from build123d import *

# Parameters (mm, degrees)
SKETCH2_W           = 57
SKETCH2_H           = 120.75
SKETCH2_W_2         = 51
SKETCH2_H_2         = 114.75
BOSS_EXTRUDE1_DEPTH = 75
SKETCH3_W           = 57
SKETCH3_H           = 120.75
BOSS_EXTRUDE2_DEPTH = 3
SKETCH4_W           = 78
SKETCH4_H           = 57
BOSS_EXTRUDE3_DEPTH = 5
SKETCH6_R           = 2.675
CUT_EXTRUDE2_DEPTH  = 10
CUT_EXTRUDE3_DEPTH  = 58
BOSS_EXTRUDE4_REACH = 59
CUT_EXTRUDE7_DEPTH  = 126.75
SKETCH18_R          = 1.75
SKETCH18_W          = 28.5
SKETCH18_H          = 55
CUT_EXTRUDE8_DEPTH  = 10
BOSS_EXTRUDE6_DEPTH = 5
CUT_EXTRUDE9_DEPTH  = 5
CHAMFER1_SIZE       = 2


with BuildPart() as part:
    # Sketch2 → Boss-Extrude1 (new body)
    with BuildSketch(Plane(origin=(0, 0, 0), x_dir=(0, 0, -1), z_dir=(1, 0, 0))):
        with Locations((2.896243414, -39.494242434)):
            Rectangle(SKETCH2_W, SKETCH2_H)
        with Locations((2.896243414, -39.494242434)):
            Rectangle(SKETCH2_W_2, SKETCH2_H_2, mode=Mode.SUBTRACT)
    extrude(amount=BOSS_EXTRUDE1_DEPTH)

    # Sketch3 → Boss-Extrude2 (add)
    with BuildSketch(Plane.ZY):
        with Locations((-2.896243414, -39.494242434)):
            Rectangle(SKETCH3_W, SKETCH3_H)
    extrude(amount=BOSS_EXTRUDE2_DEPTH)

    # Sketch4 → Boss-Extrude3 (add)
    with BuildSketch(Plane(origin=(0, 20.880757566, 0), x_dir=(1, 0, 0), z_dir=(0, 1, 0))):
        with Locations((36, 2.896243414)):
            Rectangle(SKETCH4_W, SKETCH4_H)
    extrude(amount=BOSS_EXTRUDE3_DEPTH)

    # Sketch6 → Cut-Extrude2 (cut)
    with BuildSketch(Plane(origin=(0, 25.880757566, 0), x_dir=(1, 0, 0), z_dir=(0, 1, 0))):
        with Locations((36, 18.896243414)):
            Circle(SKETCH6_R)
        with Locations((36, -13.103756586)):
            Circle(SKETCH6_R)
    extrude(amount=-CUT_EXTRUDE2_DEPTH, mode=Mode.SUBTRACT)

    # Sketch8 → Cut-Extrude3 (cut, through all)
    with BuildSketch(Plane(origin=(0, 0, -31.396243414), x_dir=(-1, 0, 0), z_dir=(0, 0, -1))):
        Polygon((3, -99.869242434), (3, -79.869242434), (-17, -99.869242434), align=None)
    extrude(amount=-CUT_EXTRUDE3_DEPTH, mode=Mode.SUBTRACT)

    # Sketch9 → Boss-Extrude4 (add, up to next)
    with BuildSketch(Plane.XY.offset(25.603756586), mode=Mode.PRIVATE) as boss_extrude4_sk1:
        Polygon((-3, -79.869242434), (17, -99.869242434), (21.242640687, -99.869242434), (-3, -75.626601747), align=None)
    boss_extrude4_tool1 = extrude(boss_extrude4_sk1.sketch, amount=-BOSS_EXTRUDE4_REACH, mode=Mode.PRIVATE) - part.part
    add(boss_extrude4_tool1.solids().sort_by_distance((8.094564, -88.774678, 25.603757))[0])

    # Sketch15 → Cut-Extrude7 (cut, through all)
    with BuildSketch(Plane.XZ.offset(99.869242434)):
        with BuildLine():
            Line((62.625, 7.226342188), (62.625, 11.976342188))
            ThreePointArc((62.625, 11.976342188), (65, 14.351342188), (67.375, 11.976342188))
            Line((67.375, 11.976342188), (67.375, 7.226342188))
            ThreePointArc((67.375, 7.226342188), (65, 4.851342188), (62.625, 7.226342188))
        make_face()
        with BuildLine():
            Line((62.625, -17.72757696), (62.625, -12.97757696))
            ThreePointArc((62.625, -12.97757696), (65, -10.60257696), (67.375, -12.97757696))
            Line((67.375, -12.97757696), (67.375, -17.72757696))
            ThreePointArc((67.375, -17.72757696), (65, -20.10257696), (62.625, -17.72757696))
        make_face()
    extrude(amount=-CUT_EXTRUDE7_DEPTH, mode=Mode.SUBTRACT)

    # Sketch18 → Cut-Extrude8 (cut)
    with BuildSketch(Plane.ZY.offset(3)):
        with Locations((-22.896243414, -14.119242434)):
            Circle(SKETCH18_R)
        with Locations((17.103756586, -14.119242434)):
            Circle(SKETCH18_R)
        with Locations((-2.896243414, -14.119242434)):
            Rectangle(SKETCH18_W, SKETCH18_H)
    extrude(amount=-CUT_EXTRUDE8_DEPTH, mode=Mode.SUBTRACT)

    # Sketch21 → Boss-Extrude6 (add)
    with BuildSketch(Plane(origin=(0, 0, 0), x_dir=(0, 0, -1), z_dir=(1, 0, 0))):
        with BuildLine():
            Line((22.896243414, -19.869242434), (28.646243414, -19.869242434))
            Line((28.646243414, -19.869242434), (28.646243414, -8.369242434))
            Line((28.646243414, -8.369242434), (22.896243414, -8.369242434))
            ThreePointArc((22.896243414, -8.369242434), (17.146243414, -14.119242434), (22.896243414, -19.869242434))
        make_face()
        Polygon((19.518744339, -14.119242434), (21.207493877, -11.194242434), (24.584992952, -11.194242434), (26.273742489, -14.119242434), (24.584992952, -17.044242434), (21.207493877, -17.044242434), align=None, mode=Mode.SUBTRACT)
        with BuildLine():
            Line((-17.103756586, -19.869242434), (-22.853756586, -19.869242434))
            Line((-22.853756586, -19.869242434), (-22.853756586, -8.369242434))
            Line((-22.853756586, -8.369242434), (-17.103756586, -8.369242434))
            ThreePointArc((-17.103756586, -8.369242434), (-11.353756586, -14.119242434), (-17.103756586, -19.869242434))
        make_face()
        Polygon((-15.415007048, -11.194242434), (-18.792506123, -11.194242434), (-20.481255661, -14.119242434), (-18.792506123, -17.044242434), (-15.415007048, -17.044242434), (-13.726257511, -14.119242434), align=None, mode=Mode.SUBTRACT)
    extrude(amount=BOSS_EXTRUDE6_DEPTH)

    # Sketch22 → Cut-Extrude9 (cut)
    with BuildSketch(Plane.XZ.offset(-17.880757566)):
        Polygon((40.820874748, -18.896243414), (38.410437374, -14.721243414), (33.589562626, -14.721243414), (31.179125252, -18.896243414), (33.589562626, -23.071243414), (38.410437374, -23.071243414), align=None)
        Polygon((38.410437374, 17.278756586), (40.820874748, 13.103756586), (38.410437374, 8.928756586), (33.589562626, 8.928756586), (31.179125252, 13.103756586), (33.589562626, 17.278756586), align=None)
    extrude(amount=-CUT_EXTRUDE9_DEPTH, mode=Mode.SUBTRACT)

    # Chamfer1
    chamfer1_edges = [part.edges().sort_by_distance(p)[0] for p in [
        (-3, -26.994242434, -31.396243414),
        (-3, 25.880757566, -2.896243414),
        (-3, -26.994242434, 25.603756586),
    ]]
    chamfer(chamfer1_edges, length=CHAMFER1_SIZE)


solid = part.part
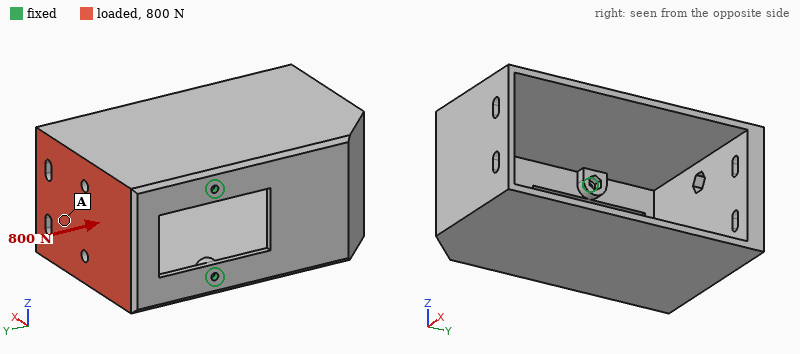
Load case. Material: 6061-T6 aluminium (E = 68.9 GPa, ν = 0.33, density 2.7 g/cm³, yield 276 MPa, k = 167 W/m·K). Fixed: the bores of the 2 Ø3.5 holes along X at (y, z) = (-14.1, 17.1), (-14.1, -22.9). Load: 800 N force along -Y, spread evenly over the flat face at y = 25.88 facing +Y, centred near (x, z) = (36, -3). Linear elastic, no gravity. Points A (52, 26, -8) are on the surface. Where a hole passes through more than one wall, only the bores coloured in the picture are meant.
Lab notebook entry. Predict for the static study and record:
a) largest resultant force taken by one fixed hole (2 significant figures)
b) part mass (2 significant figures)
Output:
400 N
300 g
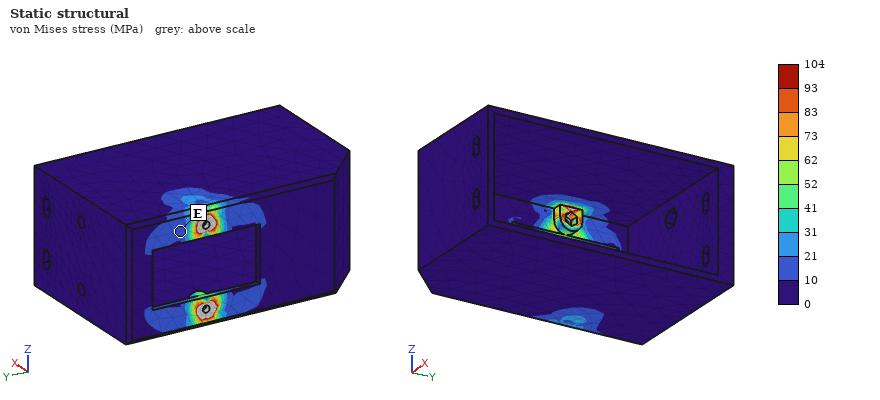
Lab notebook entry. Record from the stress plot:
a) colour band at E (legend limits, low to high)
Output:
10 to 21 MPa
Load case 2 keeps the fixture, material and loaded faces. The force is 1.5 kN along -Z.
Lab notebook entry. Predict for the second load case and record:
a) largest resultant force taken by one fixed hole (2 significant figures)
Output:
1.7 kN
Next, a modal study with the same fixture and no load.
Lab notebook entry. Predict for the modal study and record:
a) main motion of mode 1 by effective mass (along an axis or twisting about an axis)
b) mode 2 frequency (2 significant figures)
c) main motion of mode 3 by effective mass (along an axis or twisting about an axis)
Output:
along Y
710 Hz
along Z
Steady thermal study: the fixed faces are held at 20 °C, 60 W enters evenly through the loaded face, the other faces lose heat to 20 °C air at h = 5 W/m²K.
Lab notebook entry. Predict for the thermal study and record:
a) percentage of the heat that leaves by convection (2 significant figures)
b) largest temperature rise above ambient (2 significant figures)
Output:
14 %
53 K
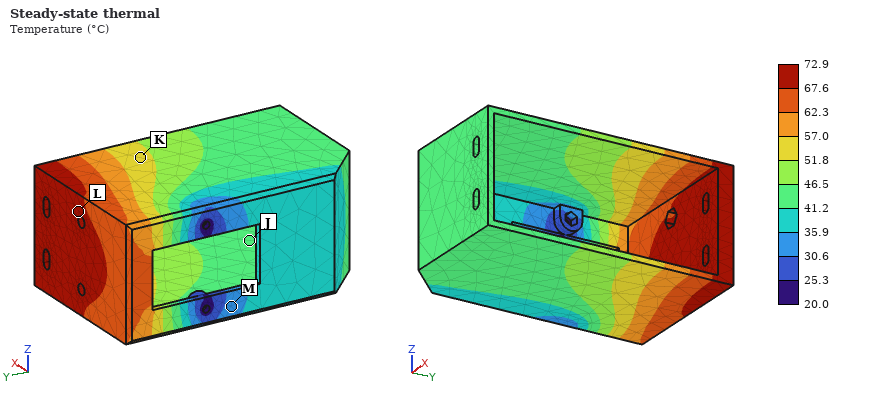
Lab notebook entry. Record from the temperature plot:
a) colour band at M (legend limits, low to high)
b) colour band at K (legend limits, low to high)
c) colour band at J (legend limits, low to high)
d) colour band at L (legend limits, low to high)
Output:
30.6 to 35.9 °C
51.8 to 57.0 °C
41.2 to 46.5 °C
67.6 to 72.9 °C
